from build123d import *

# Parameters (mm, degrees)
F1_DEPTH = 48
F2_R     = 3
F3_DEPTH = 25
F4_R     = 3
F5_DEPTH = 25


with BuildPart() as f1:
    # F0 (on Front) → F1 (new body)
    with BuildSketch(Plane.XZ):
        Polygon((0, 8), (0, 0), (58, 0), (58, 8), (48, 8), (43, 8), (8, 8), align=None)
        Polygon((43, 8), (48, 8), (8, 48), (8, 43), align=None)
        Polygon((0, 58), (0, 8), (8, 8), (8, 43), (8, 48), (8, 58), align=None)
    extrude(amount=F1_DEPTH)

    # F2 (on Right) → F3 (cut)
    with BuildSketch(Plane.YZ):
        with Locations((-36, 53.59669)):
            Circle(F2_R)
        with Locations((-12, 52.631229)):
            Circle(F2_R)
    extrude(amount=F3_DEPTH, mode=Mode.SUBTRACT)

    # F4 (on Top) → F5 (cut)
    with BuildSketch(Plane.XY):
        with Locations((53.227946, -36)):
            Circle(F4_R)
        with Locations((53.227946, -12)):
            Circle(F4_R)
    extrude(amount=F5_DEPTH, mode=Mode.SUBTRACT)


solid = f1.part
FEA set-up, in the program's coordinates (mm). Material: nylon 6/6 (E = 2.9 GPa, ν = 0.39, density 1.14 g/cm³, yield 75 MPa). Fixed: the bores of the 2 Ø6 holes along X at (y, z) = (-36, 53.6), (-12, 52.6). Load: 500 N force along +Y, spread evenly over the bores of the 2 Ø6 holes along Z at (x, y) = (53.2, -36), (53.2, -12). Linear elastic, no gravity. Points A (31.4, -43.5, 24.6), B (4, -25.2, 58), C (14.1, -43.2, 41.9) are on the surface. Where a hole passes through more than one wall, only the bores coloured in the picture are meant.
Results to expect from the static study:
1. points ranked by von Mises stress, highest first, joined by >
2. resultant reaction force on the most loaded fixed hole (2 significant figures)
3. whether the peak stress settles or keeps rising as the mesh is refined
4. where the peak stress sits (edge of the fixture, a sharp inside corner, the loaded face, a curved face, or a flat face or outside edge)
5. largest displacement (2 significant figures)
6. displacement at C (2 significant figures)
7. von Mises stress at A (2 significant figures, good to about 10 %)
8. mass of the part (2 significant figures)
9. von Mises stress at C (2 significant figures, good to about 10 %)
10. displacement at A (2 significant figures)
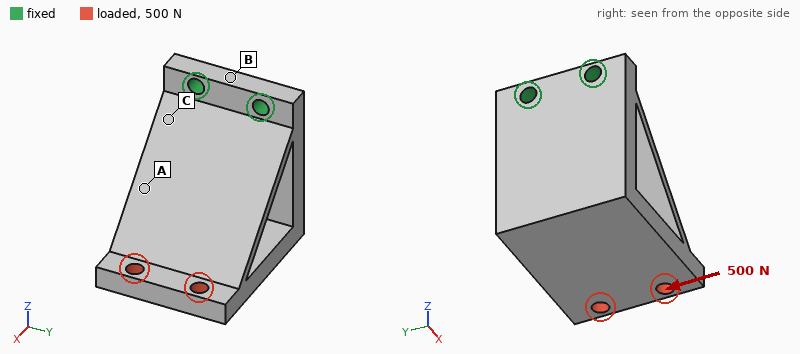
C > A > B
1.2 kN
keeps rising
edge of the fixture
1.0 mm
0.18 mm
8.4 MPa
57 g
14 MPa
0.49 mm
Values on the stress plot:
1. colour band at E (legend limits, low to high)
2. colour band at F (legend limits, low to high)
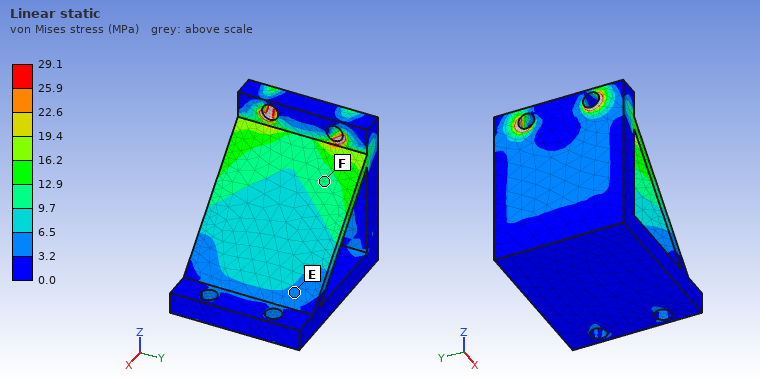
3.2 to 6.5 MPa
9.7 to 12.9 MPa
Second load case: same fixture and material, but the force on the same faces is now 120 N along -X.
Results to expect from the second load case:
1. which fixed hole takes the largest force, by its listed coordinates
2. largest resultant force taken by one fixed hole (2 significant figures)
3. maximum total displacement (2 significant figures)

(-12, 52.6)
67 N
1.0 mm
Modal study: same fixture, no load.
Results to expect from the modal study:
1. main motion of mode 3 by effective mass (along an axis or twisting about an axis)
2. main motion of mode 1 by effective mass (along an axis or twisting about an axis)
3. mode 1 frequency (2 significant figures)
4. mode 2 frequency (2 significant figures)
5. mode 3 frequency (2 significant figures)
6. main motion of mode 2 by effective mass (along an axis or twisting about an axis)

along Y
along X
320 Hz
1000 Hz
1700 Hz
along Y
